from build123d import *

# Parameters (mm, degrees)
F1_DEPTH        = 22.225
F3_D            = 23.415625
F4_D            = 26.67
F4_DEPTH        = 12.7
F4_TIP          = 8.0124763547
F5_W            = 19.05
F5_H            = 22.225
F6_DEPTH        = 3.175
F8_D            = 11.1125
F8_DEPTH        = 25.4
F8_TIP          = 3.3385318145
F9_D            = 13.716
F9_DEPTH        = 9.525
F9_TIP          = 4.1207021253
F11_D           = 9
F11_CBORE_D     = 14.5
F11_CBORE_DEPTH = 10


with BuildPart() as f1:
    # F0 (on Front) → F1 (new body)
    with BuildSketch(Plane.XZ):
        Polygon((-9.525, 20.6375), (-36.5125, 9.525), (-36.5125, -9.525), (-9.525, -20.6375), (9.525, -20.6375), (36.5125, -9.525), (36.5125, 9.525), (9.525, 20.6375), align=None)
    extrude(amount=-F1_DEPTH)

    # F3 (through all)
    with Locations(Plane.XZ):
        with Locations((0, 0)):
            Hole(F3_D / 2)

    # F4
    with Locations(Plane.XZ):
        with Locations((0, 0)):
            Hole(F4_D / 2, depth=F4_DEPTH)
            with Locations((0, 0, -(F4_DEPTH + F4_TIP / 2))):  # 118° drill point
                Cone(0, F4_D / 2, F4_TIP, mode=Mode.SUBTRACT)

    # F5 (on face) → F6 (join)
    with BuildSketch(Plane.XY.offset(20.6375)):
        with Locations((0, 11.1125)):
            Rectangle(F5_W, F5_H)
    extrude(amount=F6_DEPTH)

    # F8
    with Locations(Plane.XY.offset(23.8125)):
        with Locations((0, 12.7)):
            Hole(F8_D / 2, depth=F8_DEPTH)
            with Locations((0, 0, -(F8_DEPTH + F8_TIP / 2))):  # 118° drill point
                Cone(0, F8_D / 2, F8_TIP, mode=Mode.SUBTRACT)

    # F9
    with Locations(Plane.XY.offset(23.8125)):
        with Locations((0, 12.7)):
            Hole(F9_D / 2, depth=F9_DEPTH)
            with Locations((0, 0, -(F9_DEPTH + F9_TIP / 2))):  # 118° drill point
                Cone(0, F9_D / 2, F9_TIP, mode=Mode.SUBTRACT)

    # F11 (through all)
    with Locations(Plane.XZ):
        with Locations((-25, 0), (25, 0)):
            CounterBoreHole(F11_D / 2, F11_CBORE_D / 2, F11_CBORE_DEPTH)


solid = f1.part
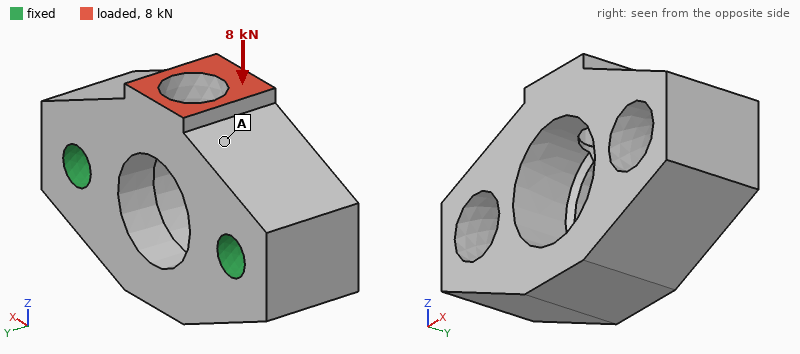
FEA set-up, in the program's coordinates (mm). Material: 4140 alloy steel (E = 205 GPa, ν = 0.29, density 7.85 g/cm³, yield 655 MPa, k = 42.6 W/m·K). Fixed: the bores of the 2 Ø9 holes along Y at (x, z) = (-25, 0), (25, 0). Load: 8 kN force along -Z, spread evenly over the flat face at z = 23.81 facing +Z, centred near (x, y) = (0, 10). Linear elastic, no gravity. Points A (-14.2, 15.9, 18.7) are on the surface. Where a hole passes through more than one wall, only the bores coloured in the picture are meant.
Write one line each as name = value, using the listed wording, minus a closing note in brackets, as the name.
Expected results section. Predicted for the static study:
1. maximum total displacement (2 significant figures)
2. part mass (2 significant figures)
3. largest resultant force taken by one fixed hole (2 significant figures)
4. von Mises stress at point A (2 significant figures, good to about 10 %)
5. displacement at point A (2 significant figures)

maximum total displacement = 13 µm
part mass = 290 g
largest resultant force taken by one fixed hole = 4.4 kN
von Mises stress at point A = 19 MPa
displacement at point A = 4.3 µm
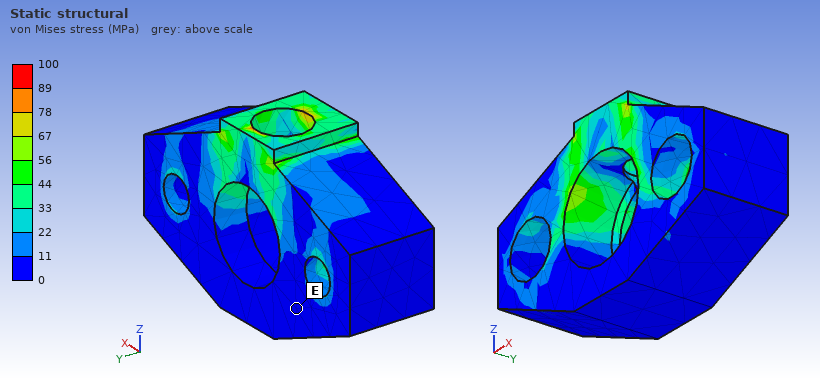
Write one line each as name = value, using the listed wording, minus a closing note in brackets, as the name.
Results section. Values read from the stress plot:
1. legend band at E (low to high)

legend band at E = 0 to 11 MPa
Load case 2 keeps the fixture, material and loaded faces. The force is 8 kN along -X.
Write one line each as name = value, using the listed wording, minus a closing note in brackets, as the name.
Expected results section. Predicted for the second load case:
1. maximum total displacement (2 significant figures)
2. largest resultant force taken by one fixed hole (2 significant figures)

maximum total displacement = 10 µm
largest resultant force taken by one fixed hole = 5.1 kN
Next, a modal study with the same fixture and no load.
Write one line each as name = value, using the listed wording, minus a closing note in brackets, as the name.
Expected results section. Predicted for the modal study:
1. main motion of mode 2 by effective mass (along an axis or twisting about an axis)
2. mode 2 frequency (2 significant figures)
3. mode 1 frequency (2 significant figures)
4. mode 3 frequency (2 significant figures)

main motion of mode 2 by effective mass = along Y
mode 2 frequency = 17 kHz
mode 1 frequency = 13 kHz
mode 3 frequency = 22 kHz
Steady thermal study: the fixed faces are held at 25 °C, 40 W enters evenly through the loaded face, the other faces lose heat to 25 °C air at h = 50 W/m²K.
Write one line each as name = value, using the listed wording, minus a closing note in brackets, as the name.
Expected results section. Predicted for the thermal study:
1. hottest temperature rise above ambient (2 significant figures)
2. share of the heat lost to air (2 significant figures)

hottest temperature rise above ambient = 62 K
share of the heat lost to air = 15 %
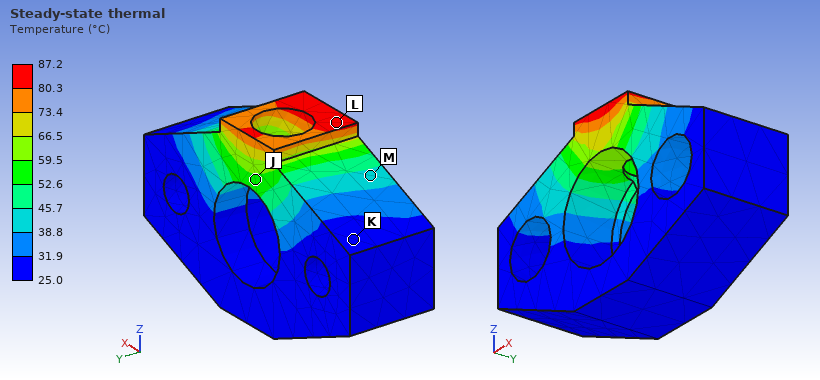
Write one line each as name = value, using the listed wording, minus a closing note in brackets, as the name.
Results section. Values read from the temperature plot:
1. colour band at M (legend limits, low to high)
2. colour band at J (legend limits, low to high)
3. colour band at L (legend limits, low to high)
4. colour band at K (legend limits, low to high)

colour band at M = 38.8 to 45.7 °C
colour band at J = 52.6 to 59.5 °C
colour band at L = 80.3 to 87.2 °C
colour band at K = 25.0 to 31.9 °C
